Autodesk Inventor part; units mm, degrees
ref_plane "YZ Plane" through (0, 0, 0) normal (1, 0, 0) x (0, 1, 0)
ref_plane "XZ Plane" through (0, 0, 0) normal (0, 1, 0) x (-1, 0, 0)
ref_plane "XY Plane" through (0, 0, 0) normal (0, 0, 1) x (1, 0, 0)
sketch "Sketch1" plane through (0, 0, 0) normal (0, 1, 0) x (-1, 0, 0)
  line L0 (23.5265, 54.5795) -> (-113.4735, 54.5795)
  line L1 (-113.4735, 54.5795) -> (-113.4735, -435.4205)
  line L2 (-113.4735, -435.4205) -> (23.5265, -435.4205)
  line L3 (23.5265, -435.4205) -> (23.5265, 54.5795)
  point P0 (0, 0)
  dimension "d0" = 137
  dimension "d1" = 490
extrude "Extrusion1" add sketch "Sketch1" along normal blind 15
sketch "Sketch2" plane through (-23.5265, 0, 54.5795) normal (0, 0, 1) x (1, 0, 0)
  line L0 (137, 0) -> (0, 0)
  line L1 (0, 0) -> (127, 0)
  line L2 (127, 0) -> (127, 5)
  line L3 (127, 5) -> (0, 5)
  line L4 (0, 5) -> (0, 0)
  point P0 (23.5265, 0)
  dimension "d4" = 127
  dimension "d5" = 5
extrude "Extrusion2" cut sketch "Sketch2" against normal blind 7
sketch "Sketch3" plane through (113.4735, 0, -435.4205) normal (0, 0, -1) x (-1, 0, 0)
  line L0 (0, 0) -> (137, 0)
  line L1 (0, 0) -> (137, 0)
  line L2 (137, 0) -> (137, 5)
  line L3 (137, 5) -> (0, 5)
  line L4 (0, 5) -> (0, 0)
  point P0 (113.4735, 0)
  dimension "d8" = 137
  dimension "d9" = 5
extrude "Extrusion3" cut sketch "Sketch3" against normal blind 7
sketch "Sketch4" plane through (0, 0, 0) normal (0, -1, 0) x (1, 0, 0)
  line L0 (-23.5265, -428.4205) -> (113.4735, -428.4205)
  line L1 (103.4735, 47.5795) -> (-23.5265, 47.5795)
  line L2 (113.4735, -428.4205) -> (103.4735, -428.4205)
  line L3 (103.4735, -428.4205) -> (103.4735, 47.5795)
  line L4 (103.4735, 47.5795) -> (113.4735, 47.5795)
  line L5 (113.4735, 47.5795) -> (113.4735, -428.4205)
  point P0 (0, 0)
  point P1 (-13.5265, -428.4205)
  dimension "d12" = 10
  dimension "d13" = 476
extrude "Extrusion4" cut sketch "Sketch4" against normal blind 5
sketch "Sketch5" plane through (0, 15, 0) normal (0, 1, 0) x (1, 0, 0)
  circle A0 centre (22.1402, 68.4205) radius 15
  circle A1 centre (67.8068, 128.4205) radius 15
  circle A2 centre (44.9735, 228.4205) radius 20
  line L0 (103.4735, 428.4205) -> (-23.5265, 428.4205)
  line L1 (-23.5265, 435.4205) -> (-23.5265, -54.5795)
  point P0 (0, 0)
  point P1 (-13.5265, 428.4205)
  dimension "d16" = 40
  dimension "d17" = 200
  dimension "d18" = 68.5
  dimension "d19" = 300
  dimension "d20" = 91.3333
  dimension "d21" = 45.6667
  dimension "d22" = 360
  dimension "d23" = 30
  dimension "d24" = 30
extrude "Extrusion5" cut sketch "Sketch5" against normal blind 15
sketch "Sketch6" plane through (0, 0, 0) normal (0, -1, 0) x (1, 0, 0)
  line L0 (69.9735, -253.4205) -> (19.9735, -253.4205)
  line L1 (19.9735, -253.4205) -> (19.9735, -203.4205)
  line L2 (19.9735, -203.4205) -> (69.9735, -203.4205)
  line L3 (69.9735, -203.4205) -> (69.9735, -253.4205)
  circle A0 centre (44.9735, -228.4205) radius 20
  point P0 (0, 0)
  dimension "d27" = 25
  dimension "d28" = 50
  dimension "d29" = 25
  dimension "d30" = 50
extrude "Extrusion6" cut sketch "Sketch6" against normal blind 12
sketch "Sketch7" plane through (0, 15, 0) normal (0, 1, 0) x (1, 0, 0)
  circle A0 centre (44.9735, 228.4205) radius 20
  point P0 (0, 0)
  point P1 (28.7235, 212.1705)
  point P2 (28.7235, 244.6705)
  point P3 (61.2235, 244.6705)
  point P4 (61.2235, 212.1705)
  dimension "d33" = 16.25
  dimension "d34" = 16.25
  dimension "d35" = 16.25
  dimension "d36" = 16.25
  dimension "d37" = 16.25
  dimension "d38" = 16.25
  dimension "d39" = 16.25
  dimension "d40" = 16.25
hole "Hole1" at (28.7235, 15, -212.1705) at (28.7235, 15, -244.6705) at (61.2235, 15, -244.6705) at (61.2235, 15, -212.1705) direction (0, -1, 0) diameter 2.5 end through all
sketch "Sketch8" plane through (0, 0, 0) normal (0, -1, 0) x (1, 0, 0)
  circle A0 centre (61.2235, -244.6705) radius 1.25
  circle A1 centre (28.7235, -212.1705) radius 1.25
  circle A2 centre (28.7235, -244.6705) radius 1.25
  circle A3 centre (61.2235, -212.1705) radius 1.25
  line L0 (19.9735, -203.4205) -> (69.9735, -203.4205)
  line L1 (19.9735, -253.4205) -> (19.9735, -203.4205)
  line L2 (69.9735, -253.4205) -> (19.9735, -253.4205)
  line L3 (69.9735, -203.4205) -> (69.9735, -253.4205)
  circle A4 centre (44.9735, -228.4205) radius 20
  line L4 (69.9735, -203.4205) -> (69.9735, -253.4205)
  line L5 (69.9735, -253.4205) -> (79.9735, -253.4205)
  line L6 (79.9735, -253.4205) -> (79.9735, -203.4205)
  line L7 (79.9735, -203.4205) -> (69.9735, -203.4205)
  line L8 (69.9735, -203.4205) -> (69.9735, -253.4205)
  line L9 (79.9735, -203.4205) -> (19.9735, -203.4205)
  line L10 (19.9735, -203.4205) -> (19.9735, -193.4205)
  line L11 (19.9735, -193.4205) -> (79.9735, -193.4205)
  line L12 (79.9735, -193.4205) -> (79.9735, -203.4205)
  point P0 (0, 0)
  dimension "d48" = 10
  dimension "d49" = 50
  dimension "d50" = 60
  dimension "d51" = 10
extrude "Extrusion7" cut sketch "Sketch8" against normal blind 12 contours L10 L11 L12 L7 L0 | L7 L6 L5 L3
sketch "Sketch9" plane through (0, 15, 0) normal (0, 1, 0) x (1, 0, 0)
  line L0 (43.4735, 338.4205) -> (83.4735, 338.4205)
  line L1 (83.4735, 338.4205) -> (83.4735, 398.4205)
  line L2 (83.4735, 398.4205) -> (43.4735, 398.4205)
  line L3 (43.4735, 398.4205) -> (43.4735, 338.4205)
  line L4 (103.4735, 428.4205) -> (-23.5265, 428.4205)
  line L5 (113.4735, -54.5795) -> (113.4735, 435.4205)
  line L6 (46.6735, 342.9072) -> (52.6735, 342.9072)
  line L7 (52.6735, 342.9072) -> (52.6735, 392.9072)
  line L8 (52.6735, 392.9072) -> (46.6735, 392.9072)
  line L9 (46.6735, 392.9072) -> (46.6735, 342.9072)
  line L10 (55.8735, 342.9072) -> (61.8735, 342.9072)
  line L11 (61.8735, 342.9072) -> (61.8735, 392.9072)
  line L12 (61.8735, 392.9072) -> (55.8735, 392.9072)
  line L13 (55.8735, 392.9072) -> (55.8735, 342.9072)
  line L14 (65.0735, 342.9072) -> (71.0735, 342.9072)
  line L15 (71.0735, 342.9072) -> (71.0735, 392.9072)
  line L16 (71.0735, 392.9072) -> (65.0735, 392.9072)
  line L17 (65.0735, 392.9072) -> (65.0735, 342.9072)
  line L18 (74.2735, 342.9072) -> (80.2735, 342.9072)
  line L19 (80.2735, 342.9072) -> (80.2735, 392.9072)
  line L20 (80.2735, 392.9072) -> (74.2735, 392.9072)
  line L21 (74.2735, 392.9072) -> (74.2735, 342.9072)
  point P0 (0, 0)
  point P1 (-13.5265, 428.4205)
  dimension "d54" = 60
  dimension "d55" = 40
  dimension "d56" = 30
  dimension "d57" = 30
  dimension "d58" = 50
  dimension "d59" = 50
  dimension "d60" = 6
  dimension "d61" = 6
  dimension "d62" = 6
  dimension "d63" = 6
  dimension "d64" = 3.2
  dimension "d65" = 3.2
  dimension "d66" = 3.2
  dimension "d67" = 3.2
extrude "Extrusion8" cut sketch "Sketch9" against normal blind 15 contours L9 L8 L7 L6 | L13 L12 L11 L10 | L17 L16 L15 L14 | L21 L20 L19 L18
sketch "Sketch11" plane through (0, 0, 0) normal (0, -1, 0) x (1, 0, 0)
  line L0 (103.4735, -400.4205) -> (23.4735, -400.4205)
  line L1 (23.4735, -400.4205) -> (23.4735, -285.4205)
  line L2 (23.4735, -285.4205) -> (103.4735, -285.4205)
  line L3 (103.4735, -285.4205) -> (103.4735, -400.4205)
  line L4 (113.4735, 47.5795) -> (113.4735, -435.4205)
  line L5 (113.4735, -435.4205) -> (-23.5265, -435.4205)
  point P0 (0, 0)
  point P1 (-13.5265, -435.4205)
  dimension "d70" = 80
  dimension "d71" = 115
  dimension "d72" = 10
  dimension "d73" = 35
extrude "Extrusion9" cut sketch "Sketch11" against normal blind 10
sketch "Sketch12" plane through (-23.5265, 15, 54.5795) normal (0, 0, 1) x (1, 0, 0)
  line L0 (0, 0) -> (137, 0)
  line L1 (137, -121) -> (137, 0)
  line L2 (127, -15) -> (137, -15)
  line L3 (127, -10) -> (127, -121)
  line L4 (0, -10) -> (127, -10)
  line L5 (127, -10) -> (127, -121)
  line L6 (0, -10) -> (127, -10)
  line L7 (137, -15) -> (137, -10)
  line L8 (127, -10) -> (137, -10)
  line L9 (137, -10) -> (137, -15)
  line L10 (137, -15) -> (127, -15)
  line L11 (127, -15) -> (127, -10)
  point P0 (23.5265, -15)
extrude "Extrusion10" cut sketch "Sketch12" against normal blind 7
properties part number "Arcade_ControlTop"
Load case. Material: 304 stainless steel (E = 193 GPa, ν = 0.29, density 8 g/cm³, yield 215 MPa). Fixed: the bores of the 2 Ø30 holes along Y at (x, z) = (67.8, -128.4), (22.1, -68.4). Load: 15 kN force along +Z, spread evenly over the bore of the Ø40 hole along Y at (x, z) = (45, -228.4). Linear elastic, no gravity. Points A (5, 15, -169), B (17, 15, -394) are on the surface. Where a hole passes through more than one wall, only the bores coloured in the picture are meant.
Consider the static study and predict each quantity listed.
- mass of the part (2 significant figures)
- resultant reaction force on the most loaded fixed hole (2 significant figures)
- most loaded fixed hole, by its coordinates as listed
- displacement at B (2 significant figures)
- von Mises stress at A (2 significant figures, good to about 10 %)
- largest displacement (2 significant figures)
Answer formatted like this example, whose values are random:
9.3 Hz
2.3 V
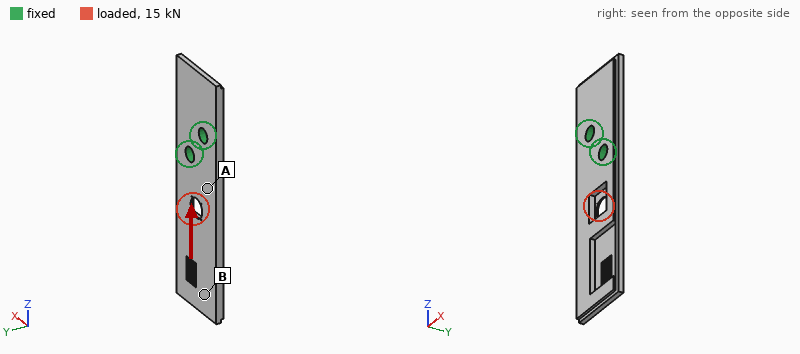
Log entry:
6.5 kg
9.5 kN
(67.8, -128.4)
0.28 mm
23 MPa
0.34 mm
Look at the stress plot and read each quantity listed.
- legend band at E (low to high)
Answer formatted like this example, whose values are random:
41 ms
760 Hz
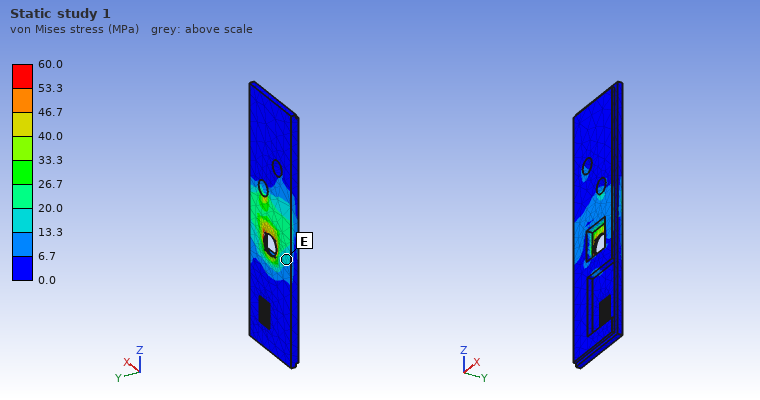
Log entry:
13.3 to 20.0 MPa
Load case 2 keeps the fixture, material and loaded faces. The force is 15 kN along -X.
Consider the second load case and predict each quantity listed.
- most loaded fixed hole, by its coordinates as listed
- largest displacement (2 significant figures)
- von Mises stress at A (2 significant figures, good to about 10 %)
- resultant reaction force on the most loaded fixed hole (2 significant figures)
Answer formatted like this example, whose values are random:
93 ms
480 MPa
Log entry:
(67.8, -128.4)
0.11 mm
19 MPa
25 kN
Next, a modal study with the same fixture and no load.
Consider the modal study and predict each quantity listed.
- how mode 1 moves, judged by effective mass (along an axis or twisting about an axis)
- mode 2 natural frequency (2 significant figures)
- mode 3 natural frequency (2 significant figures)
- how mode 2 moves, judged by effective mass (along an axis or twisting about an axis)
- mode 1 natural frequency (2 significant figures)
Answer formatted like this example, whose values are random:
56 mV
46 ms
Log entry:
along Y
470 Hz
680 Hz
twisting about Z
130 Hz
